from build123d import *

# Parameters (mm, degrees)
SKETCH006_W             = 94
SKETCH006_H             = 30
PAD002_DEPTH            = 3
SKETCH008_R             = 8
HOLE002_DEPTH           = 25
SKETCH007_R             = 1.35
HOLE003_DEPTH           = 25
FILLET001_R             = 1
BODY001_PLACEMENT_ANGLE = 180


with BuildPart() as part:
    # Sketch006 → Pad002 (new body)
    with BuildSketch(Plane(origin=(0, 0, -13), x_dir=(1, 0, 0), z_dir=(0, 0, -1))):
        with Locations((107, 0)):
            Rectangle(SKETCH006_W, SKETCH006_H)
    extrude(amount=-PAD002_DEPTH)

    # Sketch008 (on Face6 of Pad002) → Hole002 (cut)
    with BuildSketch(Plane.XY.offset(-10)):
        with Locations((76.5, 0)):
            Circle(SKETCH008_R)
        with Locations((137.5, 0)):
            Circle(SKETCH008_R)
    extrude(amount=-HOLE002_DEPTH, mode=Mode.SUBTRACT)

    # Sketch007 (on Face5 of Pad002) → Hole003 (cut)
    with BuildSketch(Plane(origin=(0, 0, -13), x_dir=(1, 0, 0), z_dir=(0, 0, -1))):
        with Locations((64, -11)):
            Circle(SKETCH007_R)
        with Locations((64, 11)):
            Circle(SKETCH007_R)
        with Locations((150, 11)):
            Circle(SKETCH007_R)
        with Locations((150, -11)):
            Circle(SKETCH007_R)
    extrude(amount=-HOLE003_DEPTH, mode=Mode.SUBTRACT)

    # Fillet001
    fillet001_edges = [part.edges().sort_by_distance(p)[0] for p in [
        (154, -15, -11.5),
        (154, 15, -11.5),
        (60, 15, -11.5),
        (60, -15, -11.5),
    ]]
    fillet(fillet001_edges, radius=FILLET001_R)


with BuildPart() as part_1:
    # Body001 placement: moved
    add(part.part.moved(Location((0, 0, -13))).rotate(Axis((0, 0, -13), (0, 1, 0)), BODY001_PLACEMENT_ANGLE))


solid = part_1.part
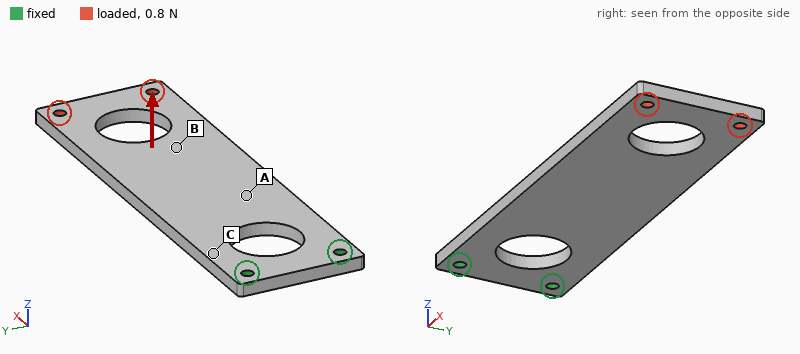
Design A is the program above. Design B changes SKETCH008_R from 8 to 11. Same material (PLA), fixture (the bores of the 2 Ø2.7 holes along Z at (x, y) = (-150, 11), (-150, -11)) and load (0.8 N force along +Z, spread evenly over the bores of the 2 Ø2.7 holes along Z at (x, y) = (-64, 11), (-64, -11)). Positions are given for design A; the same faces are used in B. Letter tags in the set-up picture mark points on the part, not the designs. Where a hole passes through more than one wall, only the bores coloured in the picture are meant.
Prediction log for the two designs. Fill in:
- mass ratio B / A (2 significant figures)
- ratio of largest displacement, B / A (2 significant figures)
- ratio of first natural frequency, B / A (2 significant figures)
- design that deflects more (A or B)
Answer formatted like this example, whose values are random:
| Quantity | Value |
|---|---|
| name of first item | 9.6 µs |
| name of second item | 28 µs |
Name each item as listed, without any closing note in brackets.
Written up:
| Quantity | Value |
|---|---|
| mass ratio B / A | 0.85 |
| ratio of largest displacement, B / A | 1.5 |
| ratio of first natural frequency, B / A | 0.90 |
| design that deflects more | B |
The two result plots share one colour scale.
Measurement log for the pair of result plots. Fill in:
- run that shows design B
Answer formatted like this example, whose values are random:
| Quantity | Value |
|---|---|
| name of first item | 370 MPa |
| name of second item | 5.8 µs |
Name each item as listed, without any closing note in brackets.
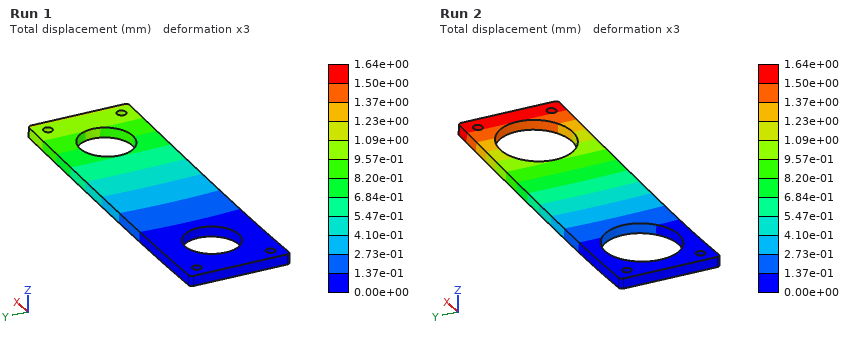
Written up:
| Quantity | Value |
|---|---|
| run that shows design B | Run 2 |
